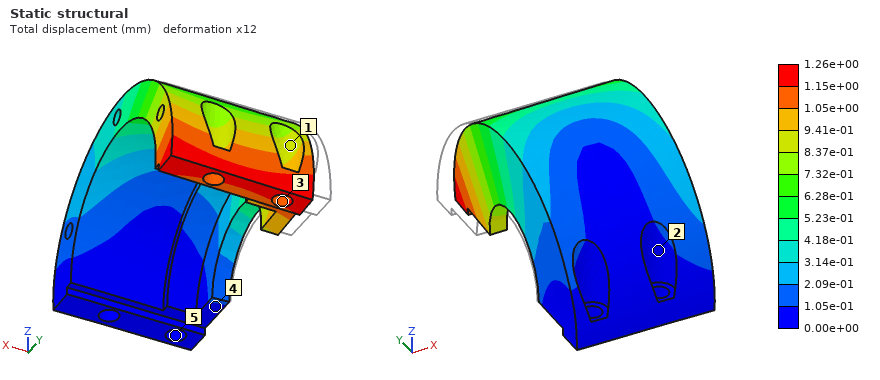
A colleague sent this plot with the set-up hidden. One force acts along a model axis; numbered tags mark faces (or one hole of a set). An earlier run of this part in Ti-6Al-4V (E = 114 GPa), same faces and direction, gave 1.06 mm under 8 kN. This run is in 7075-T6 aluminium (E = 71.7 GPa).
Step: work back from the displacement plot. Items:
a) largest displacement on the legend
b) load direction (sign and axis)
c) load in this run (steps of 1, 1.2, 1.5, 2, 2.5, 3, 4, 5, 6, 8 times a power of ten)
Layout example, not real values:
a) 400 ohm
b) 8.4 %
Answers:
a) 1.26e+00 mm
b) +X
c) 6 kN
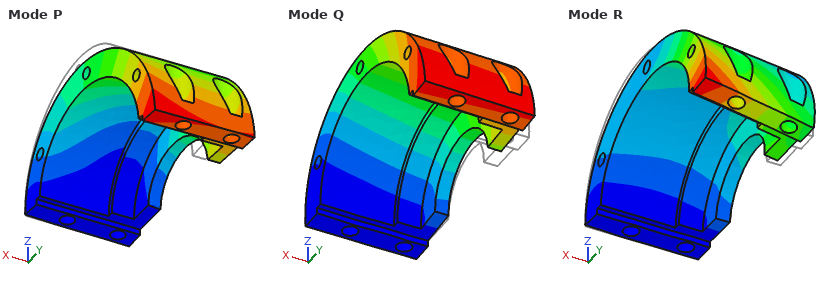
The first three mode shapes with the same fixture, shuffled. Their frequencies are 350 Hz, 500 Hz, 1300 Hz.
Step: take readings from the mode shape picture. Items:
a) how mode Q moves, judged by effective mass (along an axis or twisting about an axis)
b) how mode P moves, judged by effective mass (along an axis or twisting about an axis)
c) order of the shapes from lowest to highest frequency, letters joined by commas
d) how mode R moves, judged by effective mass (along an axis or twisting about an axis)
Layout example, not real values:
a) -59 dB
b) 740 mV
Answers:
a) along Z
b) along X
c) Q, P, R
d) along Y
